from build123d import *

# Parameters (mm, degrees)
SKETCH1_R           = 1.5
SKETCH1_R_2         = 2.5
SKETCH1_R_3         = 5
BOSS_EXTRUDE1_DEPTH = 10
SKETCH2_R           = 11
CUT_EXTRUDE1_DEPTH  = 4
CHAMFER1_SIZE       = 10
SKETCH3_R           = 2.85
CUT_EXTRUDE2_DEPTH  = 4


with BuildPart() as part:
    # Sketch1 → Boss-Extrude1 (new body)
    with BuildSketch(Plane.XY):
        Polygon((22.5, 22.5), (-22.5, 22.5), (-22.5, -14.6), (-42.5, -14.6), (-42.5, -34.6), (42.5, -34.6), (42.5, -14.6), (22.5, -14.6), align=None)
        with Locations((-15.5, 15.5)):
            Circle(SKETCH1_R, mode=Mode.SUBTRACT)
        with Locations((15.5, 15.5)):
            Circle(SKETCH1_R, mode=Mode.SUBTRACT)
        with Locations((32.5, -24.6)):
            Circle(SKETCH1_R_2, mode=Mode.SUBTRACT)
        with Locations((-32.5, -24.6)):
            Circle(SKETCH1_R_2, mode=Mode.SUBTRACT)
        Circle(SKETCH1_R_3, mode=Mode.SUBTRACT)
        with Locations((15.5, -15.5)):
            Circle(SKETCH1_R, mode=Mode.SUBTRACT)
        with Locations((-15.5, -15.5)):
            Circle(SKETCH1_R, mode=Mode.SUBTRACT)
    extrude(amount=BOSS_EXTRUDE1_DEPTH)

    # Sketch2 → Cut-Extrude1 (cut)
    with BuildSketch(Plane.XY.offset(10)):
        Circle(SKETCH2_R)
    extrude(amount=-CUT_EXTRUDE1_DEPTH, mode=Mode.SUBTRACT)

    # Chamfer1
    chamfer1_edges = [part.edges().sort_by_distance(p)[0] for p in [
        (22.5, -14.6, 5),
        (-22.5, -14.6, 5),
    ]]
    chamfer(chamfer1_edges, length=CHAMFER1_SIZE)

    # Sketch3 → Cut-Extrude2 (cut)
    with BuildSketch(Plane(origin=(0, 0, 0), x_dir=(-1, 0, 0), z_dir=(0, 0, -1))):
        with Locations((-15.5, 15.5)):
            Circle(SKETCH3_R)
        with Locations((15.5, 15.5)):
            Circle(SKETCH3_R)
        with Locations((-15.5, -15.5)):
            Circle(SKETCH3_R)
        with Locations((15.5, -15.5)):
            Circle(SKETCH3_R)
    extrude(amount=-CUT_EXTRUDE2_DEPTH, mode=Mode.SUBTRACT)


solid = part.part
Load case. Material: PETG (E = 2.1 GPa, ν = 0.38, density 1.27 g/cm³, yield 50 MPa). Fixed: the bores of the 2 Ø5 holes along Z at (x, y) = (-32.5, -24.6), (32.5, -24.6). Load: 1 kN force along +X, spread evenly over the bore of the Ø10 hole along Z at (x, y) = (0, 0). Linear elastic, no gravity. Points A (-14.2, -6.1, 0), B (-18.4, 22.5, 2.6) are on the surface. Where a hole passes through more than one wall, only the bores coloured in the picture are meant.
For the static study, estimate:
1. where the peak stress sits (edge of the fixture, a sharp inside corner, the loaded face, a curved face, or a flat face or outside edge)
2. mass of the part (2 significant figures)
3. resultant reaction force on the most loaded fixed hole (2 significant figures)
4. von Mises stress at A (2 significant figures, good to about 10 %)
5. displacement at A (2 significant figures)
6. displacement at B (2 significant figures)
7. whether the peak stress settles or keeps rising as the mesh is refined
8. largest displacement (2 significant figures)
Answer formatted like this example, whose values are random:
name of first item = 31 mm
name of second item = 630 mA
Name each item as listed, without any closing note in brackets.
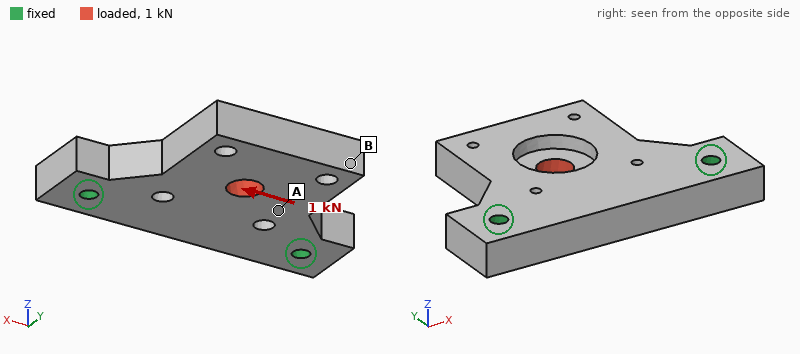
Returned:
where the peak stress sits = edge of the fixture
mass of the part = 40 g
resultant reaction force on the most loaded fixed hole = 630 N
von Mises stress at A = 6.0 MPa
displacement at A = 0.066 mm
displacement at B = 0.13 mm
whether the peak stress settles or keeps rising as the mesh is refined = keeps rising
largest displacement = 0.14 mm
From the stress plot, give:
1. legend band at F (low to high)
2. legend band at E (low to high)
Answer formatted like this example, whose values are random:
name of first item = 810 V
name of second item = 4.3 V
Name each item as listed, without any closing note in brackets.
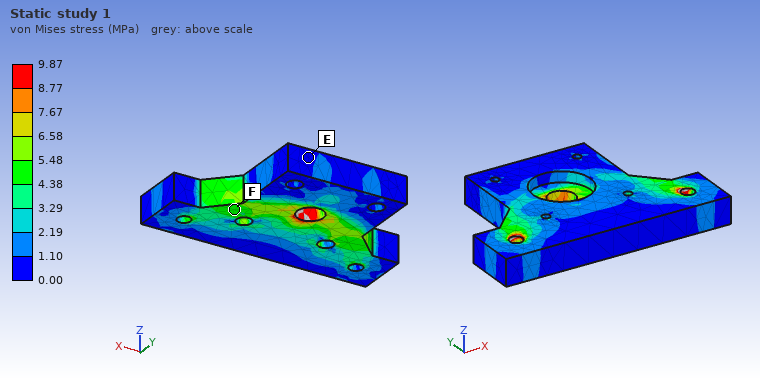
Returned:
legend band at F = 4.38 to 5.48 MPa
legend band at E = 0.00 to 1.10 MPa
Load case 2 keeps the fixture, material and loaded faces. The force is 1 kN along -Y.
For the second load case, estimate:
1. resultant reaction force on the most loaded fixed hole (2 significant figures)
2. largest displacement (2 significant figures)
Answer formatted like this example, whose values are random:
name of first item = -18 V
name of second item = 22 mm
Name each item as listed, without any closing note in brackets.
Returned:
resultant reaction force on the most loaded fixed hole = 560 N
largest displacement = 0.36 mm
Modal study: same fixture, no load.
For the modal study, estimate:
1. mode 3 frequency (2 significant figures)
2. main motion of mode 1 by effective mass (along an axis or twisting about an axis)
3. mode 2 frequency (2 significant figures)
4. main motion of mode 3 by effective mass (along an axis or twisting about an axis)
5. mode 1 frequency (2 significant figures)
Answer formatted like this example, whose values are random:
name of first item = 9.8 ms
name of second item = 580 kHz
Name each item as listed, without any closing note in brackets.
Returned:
mode 3 frequency = 2600 Hz
main motion of mode 1 by effective mass = along Z
mode 2 frequency = 2000 Hz
main motion of mode 3 by effective mass = along Z
mode 1 frequency = 710 Hz
